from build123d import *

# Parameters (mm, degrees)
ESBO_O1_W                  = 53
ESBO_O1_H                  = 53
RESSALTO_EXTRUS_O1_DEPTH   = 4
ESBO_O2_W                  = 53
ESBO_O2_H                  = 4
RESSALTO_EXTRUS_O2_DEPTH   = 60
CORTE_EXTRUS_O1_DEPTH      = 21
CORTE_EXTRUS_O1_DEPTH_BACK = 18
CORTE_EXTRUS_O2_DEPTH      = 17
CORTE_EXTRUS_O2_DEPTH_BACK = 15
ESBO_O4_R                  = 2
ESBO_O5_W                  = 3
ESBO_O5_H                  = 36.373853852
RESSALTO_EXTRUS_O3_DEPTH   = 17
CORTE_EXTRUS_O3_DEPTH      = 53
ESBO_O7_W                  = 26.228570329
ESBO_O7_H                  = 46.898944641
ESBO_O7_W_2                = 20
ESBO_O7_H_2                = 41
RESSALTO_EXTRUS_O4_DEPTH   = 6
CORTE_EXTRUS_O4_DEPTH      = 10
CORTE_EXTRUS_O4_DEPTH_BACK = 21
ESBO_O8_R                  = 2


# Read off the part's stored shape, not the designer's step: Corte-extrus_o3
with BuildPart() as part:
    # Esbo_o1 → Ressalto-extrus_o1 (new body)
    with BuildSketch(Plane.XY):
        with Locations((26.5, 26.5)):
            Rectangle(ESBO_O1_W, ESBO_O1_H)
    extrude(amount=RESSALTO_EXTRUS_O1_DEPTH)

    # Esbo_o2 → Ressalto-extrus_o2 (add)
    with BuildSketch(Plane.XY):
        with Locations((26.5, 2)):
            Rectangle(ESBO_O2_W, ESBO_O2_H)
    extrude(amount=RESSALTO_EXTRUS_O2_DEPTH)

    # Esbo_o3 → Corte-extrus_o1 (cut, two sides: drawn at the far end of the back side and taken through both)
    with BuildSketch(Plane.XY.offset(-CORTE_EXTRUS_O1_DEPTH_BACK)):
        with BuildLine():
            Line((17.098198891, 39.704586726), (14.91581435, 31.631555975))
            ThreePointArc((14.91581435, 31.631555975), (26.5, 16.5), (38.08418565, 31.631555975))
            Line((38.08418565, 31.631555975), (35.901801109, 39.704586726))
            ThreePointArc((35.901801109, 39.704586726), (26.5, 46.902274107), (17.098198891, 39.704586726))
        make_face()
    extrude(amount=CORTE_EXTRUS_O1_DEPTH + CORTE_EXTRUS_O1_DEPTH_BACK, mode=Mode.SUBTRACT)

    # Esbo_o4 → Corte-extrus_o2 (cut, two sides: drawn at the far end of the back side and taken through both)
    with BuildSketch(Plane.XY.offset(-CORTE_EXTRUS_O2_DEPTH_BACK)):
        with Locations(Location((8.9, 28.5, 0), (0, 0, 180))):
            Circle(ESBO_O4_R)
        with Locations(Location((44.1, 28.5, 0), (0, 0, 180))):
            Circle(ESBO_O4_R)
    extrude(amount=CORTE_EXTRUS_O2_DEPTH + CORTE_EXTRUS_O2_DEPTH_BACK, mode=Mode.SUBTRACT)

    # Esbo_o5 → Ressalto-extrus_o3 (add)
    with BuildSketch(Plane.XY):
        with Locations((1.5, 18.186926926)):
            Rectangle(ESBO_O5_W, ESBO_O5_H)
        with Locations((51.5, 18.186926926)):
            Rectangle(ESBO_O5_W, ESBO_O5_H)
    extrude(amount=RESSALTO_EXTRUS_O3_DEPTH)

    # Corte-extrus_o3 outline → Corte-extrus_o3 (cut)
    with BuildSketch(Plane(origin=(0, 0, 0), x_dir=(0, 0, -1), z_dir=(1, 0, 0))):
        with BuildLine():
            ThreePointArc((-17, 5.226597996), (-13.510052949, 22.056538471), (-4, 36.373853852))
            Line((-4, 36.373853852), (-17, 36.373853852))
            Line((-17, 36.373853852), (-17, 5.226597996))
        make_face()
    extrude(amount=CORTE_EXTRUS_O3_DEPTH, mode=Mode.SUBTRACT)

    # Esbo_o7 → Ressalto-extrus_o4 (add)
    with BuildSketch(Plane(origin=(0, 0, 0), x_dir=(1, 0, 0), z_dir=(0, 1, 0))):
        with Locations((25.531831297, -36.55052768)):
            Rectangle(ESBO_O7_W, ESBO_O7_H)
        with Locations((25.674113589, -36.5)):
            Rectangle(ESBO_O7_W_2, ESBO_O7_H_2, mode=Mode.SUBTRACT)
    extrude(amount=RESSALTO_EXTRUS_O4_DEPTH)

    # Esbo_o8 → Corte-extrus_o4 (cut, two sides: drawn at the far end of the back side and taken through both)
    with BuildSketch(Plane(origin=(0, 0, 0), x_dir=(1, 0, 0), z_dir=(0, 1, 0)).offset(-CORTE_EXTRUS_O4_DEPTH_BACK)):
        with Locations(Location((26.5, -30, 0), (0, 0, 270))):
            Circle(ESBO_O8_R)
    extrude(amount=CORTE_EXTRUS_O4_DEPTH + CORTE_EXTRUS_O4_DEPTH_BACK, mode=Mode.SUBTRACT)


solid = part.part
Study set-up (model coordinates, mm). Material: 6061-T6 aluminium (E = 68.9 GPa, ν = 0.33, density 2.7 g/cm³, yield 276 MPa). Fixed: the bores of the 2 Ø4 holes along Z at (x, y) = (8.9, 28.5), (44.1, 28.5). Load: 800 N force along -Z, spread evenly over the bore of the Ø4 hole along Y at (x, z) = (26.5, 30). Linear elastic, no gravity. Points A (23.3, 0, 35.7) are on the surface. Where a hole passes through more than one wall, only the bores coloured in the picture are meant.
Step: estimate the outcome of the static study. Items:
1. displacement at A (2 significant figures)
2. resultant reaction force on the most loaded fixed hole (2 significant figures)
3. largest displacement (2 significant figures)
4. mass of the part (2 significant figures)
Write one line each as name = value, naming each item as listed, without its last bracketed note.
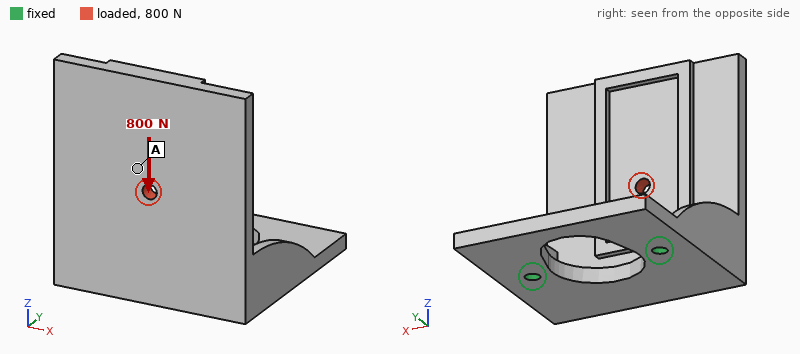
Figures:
displacement at A = 0.30 mm
resultant reaction force on the most loaded fixed hole = 430 N
largest displacement = 0.45 mm
mass of the part = 63 g
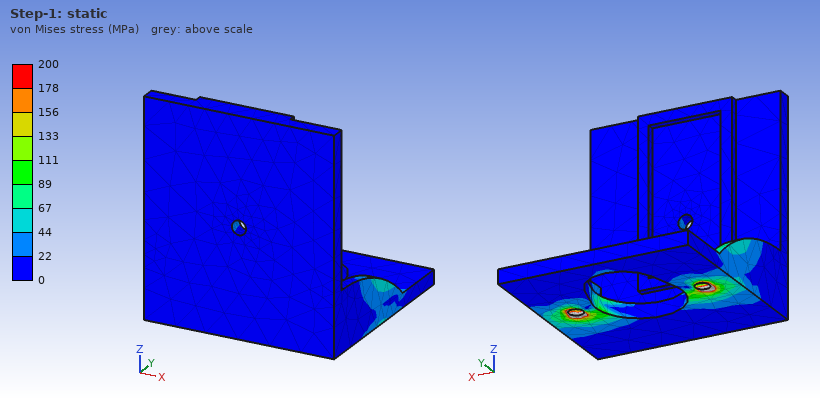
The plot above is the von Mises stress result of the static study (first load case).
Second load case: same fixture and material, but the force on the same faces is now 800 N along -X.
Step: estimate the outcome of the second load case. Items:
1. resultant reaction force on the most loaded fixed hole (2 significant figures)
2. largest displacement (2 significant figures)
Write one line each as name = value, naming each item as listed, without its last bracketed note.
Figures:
resultant reaction force on the most loaded fixed hole = 810 N
largest displacement = 0.37 mm
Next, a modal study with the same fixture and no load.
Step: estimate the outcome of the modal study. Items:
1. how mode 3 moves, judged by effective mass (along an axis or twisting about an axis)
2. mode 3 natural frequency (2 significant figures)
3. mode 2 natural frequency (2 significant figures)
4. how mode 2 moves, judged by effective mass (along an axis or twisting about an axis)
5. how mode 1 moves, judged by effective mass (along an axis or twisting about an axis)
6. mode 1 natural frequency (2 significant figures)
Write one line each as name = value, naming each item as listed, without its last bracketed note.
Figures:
how mode 3 moves, judged by effective mass = along Z
mode 3 natural frequency = 2300 Hz
mode 2 natural frequency = 1400 Hz
how mode 2 moves, judged by effective mass = along X
how mode 1 moves, judged by effective mass = along Y
mode 1 natural frequency = 840 Hz
